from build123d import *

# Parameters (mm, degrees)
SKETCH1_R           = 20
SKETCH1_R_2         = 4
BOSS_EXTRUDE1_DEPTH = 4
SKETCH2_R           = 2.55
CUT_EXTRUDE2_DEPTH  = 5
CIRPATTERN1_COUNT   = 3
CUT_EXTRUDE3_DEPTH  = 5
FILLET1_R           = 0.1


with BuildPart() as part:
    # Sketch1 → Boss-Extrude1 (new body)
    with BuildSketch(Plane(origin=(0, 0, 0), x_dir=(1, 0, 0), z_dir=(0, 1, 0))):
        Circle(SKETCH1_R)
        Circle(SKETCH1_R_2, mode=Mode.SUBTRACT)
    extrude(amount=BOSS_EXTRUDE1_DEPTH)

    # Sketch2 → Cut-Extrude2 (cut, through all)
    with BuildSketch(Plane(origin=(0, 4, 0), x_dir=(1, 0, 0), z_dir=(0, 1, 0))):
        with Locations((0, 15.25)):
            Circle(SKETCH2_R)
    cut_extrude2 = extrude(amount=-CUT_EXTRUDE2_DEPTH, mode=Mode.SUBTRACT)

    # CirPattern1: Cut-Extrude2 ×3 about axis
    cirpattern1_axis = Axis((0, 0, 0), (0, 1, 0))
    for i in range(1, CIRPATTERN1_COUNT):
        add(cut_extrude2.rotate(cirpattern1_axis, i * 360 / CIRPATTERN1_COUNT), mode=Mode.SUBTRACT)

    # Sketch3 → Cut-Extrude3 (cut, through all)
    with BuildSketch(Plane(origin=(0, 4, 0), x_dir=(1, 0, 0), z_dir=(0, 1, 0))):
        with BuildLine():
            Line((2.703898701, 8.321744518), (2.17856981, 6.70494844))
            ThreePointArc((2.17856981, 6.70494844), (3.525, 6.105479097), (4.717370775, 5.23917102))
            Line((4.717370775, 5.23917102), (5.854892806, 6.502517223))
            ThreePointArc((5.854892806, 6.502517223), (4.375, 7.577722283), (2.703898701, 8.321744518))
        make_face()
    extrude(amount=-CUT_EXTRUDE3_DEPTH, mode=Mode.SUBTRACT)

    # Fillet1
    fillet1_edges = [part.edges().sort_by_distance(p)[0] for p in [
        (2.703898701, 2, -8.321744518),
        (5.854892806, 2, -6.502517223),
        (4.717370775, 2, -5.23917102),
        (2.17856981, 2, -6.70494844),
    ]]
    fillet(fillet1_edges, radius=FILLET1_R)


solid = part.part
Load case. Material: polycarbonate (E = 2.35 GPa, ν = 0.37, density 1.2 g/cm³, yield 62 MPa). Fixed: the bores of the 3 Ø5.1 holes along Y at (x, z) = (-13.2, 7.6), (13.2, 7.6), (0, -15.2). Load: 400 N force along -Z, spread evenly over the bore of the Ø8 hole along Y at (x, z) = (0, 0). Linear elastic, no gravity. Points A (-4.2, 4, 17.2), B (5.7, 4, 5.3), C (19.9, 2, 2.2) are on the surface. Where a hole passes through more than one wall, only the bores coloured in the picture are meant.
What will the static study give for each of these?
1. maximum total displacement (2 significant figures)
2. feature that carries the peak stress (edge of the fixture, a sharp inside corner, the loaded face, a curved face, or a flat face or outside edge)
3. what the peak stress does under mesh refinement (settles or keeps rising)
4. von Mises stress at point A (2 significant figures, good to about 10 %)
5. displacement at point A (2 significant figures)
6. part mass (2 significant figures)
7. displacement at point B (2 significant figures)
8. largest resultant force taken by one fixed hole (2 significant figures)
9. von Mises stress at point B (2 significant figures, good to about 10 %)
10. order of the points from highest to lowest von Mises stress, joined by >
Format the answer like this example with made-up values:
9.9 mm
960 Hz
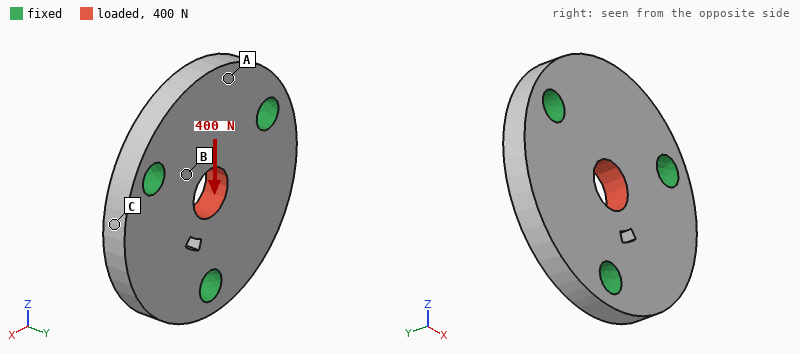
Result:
27 µm
a sharp inside corner
keeps rising
1.7 MPa
14 µm
5.5 g
15 µm
140 N
2.9 MPa
B > A > C
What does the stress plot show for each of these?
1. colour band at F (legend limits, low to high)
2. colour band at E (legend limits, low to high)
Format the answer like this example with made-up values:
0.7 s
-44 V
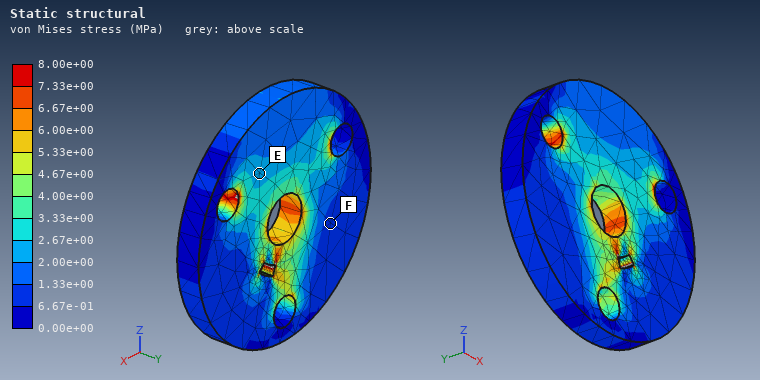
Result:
6.67e-01 to 1.33e+00 MPa
2.00e+00 to 2.67e+00 MPa
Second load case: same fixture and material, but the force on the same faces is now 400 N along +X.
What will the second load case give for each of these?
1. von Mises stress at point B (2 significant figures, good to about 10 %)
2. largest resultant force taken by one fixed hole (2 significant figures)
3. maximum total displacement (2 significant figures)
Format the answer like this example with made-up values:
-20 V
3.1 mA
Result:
3.6 MPa
140 N
27 µm
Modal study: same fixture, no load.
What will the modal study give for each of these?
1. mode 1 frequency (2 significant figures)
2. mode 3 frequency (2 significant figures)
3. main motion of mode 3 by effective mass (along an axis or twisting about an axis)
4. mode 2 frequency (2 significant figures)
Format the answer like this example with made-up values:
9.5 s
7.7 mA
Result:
5600 Hz
5900 Hz
along Y
5600 Hz
